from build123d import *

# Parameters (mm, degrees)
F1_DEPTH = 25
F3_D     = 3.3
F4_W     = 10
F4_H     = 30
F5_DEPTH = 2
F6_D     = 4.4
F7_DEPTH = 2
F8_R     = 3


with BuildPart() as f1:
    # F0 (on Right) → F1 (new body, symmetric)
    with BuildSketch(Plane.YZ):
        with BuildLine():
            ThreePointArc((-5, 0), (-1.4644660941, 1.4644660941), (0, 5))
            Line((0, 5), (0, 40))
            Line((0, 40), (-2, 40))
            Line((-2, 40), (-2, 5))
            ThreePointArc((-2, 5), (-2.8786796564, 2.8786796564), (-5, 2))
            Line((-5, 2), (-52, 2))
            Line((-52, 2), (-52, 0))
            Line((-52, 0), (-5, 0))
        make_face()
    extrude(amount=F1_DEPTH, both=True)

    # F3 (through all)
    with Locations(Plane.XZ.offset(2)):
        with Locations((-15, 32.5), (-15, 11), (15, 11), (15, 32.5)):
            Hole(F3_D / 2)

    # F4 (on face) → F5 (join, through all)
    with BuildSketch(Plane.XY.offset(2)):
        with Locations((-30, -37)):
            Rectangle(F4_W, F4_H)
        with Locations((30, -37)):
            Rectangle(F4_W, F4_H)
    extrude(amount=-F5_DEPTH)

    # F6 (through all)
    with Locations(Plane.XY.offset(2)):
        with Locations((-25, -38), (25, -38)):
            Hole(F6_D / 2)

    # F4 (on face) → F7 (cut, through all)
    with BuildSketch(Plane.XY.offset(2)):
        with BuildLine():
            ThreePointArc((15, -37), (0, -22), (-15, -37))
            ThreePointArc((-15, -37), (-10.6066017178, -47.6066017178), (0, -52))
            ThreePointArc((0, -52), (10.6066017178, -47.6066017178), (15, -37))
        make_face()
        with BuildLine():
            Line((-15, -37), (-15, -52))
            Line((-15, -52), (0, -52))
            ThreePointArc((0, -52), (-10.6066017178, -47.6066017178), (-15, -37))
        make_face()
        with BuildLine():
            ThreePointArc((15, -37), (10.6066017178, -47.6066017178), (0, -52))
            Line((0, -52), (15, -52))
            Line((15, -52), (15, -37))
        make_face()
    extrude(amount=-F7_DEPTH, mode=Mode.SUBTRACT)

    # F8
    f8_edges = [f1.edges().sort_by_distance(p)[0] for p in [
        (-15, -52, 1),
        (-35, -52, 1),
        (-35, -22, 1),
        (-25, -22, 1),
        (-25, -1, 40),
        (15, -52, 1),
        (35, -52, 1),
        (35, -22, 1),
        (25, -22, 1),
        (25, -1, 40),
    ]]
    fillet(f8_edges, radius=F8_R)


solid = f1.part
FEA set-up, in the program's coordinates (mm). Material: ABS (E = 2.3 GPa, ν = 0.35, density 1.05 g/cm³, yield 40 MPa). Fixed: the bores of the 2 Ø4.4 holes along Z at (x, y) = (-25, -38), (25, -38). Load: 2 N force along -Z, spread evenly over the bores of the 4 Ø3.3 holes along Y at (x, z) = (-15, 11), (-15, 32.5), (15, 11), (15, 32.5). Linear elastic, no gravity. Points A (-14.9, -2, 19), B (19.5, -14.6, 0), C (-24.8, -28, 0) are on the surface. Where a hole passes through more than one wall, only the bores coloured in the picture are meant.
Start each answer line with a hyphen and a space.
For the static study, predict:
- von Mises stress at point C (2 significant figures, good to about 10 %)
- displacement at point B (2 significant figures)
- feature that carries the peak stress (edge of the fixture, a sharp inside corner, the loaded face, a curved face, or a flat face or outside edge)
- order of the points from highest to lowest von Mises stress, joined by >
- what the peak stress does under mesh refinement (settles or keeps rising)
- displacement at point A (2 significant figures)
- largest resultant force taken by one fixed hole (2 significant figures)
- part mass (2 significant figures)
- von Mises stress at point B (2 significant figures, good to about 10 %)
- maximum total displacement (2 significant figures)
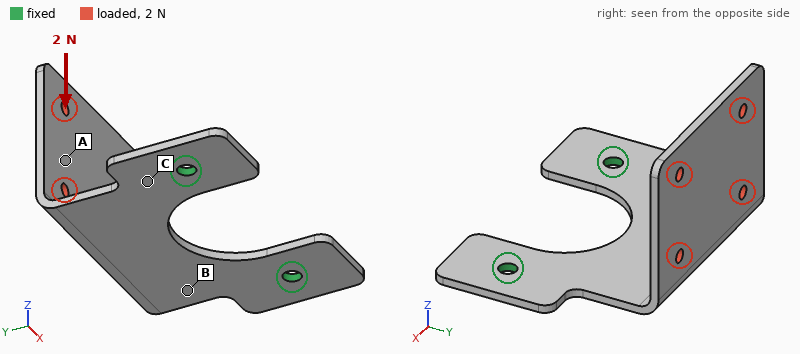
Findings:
- 1.9 MPa
- 0.26 mm
- edge of the fixture
- C > B > A
- keeps rising
- 0.66 mm
- 1.0 N
- 8.7 g
- 1.2 MPa
- 1.0 mm
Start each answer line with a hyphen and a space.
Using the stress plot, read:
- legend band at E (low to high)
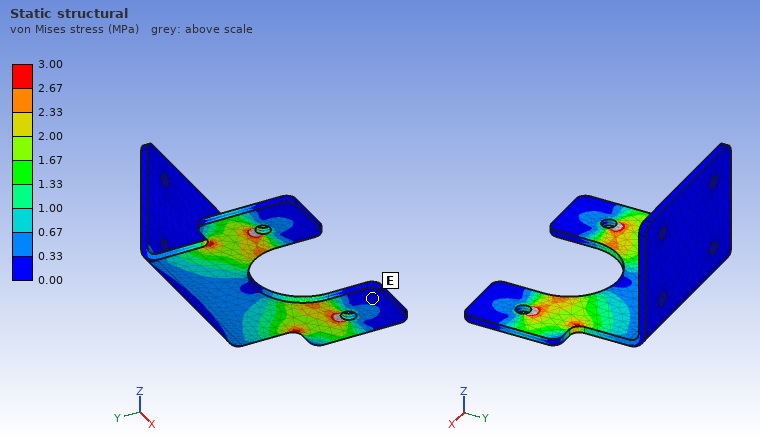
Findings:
- 0.00 to 0.33 MPa
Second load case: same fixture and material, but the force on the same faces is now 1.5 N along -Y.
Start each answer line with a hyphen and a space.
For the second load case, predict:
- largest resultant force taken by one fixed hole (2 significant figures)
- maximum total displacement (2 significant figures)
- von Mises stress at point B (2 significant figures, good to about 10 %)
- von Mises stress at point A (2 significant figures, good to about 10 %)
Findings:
- 0.86 N
- 0.87 mm
- 1.1 MPa
- 0.27 MPa
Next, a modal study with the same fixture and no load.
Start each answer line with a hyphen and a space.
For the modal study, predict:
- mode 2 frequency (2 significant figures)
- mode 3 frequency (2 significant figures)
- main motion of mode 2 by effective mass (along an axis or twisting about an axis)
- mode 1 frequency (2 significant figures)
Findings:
- 230 Hz
- 310 Hz
- along X
- 100 Hz
